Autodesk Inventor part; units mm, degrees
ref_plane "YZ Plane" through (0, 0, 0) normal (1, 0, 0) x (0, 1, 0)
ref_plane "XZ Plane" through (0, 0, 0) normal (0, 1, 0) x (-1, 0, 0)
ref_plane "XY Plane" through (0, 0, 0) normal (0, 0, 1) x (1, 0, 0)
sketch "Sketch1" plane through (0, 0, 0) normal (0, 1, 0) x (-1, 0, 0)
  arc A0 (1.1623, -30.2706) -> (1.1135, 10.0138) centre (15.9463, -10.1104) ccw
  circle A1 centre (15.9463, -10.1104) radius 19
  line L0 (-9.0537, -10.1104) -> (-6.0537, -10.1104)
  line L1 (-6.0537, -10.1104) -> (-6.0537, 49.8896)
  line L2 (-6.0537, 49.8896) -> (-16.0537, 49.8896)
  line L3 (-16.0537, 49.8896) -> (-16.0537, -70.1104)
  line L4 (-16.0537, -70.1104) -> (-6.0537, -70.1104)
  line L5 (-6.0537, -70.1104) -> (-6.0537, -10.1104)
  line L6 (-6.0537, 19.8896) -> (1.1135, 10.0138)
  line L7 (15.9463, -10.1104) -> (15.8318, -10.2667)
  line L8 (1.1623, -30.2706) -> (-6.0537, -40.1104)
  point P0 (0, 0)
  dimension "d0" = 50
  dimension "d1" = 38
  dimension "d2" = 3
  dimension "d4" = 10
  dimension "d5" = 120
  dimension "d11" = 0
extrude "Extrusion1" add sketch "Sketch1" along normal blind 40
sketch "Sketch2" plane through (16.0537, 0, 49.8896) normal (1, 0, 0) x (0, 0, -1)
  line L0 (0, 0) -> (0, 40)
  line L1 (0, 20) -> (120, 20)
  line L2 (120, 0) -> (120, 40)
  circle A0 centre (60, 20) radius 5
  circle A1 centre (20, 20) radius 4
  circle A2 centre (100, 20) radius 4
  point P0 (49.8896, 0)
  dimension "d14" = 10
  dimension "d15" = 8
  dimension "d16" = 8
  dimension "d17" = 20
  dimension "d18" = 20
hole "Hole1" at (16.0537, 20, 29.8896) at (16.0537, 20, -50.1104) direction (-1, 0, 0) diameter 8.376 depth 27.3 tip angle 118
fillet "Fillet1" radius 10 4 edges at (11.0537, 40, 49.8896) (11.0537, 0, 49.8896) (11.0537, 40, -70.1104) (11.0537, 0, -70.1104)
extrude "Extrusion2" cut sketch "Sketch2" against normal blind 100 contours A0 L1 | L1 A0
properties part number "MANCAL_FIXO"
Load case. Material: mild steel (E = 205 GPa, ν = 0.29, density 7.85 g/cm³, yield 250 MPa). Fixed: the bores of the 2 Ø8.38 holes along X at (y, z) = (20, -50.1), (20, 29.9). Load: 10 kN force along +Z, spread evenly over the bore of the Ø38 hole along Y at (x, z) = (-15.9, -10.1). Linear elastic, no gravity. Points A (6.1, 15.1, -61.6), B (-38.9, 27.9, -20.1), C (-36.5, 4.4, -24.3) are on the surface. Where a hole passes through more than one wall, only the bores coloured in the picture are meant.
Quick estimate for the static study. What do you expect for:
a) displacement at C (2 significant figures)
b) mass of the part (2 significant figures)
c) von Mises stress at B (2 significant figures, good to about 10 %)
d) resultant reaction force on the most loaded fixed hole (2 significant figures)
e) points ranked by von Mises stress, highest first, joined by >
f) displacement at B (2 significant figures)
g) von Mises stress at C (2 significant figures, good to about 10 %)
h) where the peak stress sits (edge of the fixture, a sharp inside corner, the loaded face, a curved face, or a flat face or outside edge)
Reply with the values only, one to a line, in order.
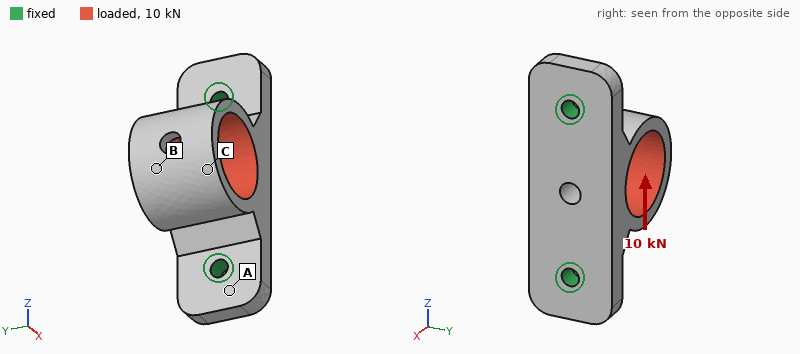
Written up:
77 µm
630 g
46 MPa
6.4 kN
C > B > A
77 µm
64 MPa
the loaded face
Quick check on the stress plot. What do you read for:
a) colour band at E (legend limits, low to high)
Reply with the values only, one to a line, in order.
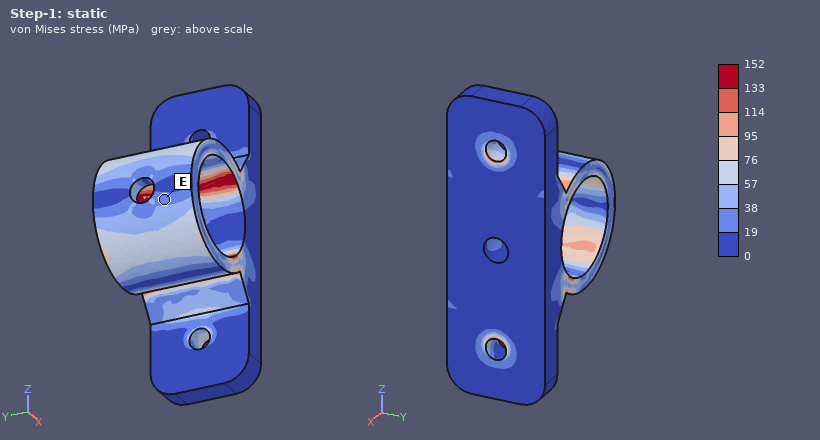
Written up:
19 to 38 MPa
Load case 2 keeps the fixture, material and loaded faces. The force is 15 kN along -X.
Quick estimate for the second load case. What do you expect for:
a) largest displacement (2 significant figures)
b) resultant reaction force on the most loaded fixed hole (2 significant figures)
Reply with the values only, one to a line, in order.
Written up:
28 µm
8.5 kN
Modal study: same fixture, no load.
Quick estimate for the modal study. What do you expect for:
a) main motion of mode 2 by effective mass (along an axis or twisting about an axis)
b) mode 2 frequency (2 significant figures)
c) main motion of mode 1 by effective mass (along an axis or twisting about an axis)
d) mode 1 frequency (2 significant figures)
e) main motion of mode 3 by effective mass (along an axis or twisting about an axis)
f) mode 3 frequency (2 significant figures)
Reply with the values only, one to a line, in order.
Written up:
along Z
3900 Hz
along Y
3000 Hz
along X
6200 Hz
